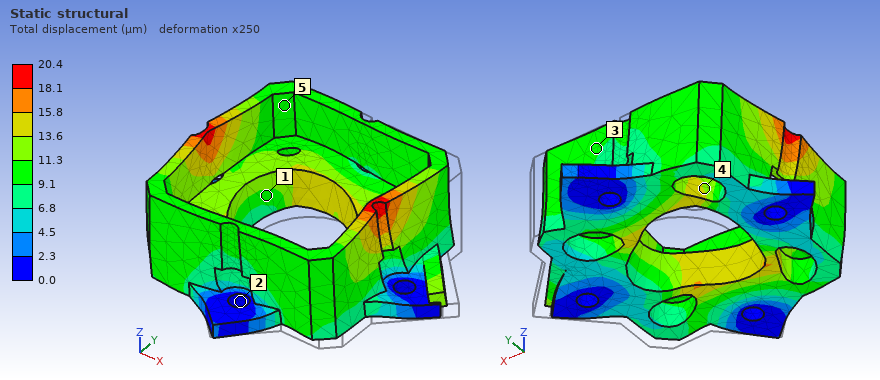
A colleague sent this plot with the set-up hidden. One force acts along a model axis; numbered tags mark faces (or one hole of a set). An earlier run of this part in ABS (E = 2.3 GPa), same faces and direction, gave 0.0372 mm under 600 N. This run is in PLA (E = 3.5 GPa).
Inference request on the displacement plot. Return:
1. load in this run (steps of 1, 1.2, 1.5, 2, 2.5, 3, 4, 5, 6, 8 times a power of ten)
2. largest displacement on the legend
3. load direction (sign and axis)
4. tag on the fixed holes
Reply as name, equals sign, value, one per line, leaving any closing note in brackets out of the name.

load in this run = 500 N
largest displacement on the legend = 20.4 µm
load direction = -X
tag on the fixed holes = 2
